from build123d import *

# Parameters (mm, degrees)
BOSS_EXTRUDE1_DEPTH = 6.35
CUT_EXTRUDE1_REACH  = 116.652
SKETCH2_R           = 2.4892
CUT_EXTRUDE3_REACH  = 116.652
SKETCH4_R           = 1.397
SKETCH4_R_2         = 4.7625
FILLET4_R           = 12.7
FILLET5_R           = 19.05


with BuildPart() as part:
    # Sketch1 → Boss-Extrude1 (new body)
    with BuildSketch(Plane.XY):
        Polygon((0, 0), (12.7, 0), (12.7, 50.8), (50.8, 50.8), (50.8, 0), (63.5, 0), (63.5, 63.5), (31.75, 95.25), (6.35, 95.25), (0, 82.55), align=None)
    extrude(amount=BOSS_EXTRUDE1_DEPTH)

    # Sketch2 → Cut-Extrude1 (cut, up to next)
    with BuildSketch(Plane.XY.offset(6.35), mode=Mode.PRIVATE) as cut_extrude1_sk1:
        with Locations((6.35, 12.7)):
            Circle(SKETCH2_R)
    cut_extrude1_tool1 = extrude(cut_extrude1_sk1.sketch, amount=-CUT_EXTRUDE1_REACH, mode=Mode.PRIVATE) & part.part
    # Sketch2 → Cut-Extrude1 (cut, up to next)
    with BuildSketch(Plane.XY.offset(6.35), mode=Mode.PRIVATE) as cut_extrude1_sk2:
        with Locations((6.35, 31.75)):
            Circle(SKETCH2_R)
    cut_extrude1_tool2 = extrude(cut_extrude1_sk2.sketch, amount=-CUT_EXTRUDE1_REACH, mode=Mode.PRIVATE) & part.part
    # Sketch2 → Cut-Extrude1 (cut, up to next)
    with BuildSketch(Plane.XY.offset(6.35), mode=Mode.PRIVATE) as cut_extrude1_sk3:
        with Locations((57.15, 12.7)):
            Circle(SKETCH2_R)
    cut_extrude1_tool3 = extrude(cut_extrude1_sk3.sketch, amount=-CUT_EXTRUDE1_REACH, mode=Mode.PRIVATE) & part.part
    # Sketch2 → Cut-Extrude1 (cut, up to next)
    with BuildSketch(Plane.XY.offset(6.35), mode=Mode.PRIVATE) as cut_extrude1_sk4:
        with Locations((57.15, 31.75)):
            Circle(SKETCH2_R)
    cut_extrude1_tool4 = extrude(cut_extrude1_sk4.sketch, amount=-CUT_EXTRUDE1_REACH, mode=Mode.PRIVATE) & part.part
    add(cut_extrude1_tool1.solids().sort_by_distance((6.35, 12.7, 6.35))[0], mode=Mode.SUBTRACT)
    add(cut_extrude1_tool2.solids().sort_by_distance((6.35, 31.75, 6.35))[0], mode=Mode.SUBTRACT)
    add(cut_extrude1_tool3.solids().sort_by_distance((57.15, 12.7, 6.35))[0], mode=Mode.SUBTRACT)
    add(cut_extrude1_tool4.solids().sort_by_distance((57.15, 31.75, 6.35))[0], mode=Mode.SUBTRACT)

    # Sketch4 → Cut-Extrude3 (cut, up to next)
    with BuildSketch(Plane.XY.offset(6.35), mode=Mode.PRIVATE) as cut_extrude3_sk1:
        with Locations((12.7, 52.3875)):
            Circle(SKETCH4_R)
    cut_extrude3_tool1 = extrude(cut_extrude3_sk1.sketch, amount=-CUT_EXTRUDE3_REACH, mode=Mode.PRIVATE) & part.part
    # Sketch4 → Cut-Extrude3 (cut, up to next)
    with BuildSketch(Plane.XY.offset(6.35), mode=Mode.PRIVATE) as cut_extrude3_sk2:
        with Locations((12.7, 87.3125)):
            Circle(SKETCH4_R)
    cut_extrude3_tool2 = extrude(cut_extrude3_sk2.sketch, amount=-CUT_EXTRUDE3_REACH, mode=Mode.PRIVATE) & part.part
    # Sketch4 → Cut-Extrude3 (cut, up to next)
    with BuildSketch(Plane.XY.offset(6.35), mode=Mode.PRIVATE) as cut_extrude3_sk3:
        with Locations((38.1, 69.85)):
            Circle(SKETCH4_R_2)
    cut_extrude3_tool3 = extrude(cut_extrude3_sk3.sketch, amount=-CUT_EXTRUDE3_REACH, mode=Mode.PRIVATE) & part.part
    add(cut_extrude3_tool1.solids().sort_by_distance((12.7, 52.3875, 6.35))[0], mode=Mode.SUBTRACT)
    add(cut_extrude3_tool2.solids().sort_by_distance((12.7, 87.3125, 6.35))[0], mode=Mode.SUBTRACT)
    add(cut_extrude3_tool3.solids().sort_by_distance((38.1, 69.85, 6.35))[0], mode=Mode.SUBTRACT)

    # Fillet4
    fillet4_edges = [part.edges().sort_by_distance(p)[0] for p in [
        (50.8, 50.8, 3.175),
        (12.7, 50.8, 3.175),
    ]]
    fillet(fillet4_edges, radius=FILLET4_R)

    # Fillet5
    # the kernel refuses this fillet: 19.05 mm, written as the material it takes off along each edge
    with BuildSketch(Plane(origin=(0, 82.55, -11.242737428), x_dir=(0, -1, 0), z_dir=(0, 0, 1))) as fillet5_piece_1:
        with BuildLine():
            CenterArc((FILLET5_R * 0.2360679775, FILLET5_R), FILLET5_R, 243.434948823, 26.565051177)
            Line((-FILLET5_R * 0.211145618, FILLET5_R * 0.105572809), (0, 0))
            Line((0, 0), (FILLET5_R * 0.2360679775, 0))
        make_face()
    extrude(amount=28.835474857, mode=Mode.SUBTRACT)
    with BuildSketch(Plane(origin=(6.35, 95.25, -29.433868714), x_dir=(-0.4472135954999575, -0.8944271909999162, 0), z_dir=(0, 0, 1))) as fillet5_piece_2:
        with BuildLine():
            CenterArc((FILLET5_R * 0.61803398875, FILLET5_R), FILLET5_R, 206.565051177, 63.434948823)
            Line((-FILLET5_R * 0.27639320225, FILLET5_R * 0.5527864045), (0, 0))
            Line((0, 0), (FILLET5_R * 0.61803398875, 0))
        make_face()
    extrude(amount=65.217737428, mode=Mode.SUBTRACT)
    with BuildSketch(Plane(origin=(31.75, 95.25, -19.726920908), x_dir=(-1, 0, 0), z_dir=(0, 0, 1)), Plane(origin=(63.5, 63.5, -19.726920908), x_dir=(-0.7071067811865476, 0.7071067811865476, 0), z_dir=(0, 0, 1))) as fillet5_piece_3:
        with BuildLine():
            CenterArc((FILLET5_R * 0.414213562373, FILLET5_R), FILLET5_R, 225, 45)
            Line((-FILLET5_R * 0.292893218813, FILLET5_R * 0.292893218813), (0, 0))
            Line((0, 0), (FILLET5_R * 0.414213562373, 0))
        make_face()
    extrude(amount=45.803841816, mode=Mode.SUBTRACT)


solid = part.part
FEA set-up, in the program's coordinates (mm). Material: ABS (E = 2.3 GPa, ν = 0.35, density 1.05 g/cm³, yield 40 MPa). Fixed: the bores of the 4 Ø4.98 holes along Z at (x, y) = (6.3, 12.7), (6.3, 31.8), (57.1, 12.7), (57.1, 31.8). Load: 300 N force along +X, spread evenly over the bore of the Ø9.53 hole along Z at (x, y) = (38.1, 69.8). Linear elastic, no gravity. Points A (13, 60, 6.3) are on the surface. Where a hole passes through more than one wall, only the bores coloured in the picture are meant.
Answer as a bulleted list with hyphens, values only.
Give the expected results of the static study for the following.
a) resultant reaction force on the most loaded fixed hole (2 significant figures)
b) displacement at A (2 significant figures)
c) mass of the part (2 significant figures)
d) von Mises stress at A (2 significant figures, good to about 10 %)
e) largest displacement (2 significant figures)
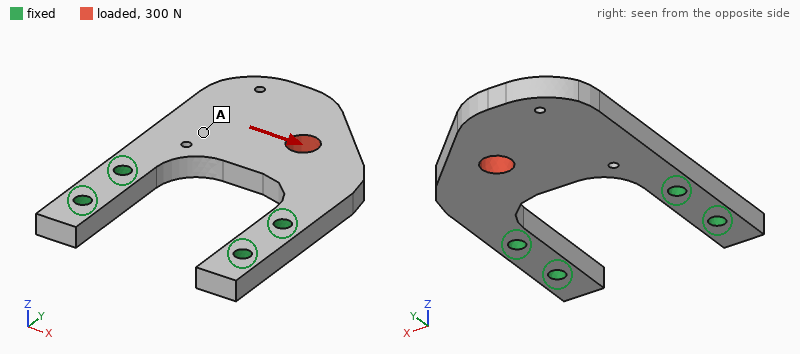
- 240 N
- 0.11 mm
- 23 g
- 1.3 MPa
- 0.15 mm
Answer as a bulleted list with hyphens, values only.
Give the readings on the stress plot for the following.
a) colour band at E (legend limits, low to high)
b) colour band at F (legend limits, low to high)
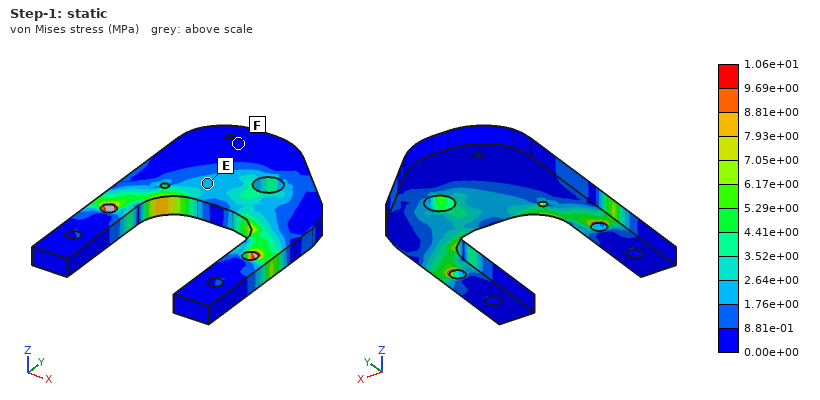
- 1.76e+00 to 2.64e+00 MPa
- 0.00e+00 to 8.81e-01 MPa
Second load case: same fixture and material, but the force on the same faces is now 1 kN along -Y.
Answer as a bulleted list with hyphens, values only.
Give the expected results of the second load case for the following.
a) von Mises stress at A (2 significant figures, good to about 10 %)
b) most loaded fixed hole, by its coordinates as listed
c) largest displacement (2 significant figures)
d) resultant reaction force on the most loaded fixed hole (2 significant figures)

- 3.0 MPa
- (57.1, 31.8)
- 0.16 mm
- 610 N
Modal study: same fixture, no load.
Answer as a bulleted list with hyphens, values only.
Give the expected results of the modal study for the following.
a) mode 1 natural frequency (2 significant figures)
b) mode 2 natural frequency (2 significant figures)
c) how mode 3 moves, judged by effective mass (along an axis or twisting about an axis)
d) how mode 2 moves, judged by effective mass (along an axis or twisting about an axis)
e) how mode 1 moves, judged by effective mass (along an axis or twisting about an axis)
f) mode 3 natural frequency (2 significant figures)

- 330 Hz
- 1200 Hz
- along X
- twisting about Y
- along Z
- 2000 Hz
